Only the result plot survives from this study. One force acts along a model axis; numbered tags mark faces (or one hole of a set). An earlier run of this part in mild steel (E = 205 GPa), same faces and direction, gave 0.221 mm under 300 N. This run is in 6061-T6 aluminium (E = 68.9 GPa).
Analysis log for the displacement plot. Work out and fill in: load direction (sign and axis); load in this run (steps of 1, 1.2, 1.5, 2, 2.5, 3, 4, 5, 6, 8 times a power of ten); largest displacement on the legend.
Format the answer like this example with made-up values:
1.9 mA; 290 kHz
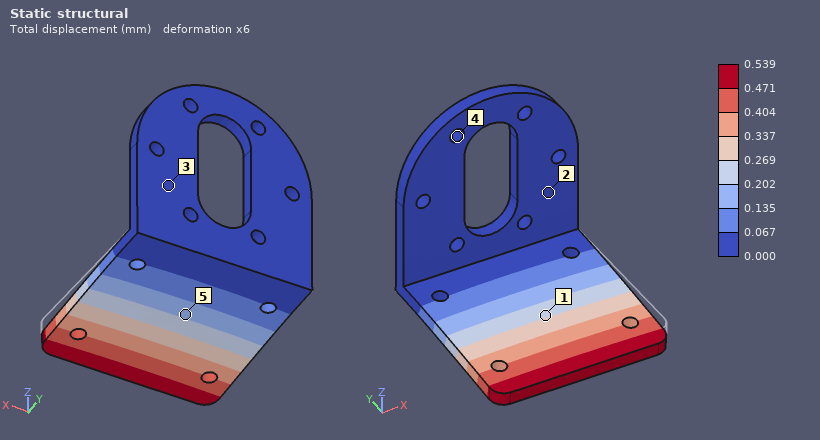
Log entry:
-Z; 250 N; 0.539 mm
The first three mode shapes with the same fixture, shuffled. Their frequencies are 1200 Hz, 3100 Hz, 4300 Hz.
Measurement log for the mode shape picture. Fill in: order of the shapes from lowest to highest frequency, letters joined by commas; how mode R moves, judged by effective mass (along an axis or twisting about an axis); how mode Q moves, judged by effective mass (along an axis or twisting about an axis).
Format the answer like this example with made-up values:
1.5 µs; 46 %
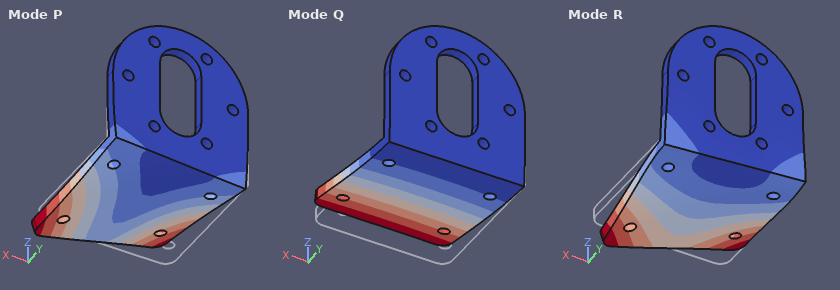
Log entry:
Q, P, R; along X; along Z
